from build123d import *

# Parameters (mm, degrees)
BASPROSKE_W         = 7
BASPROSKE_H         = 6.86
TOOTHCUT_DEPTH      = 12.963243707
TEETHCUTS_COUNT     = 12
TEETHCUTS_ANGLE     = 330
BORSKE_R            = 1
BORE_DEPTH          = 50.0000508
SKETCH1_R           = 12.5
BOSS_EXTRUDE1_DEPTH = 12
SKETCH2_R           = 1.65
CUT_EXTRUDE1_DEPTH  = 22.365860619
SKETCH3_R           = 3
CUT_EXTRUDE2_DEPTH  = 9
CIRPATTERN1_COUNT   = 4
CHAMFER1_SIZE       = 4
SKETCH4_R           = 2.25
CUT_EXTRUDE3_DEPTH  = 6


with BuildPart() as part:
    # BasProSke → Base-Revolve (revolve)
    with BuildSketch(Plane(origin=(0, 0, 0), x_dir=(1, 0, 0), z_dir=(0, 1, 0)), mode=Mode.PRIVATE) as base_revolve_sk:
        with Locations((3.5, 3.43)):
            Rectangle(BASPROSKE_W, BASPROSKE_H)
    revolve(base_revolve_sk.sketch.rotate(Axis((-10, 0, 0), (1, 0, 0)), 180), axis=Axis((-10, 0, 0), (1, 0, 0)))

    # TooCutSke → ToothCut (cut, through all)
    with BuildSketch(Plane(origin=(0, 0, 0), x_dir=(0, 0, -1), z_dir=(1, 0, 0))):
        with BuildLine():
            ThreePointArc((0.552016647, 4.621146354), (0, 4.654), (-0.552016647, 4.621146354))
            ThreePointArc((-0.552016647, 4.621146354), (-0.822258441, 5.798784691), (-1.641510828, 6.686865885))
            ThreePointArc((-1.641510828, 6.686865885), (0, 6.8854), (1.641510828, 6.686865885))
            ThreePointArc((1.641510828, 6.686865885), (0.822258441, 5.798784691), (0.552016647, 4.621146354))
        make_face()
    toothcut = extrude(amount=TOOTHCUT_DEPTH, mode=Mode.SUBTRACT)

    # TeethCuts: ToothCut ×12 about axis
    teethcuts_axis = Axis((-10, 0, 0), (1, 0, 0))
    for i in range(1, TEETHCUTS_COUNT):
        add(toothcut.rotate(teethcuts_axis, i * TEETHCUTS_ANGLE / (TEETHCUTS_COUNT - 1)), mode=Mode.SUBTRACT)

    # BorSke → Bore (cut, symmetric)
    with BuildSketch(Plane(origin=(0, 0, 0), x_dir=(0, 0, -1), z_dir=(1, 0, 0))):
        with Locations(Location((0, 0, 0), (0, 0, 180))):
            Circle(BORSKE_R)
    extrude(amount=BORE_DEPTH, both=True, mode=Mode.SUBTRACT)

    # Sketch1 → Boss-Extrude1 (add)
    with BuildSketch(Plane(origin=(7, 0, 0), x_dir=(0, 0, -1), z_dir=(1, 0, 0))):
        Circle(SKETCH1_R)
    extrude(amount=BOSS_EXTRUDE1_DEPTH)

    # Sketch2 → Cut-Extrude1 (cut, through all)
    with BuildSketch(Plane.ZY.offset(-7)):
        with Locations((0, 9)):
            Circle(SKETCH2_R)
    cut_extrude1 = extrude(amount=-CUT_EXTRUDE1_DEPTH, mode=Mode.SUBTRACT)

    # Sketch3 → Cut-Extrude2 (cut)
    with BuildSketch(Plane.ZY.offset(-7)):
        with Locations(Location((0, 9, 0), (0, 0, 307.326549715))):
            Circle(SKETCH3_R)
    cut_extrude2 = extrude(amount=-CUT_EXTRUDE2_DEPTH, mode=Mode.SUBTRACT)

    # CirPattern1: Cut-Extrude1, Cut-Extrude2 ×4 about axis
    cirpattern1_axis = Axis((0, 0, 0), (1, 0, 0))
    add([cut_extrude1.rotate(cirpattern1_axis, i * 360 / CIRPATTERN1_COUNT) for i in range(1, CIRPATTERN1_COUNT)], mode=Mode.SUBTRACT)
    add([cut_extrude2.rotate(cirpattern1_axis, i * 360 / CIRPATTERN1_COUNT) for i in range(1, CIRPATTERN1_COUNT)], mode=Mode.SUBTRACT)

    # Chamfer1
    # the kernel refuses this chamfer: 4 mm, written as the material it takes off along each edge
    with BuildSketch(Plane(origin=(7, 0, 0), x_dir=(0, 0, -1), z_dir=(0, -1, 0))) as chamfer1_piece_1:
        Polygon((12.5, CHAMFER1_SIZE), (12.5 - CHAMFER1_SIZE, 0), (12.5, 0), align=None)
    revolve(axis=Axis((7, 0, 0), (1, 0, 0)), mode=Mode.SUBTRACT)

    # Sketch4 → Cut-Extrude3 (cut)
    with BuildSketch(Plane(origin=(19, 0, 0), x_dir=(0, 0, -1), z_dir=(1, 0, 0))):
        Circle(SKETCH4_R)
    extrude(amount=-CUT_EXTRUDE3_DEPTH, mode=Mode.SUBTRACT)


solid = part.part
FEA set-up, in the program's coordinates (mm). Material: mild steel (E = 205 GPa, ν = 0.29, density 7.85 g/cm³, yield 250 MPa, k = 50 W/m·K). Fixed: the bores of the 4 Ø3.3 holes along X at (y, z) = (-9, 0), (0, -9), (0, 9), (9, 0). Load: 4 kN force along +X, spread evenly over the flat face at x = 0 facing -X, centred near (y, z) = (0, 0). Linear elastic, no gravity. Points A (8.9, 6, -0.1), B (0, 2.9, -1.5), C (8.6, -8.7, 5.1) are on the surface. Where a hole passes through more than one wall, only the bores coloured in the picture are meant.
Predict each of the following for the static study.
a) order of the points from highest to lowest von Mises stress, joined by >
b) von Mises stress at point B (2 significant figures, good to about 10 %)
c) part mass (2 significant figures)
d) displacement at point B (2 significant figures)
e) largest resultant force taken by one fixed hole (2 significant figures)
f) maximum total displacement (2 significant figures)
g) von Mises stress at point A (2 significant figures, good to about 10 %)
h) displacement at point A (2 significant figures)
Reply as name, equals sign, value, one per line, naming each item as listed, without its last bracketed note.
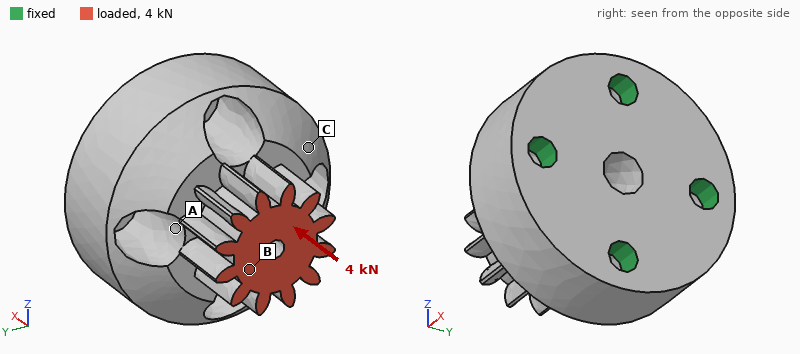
order of the points from highest to lowest von Mises stress, joined by > = B > A > C
von Mises stress at point B = 41 MPa
part mass = 39 g
displacement at point B = 3.5 µm
largest resultant force taken by one fixed hole = 1.0 kN
maximum total displacement = 3.6 µm
von Mises stress at point A = 21 MPa
displacement at point A = 1.9 µm
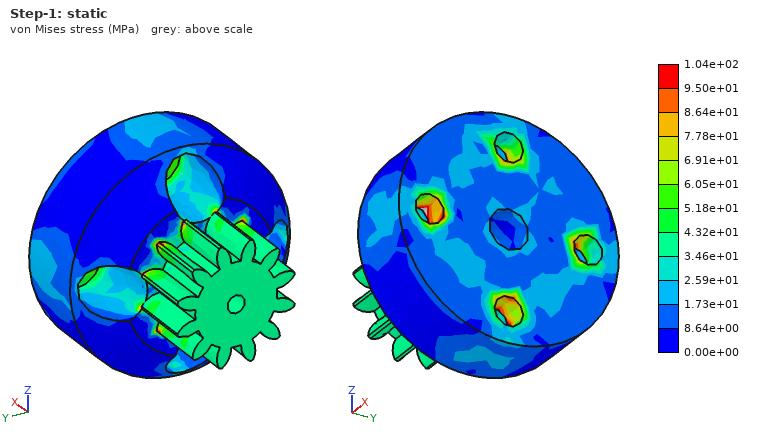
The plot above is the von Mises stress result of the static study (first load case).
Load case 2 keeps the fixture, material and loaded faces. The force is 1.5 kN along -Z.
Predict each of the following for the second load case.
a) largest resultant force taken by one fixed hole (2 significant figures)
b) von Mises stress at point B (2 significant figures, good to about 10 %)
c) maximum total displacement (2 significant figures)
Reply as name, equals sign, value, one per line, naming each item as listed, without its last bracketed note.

largest resultant force taken by one fixed hole = 1.4 kN
von Mises stress at point B = 32 MPa
maximum total displacement = 10.0 µm
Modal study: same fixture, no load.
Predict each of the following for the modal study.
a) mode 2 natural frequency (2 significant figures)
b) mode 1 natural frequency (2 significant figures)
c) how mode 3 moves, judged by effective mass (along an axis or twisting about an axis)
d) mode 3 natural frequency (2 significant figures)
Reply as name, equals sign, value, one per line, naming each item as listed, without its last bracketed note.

mode 2 natural frequency = 29 kHz
mode 1 natural frequency = 29 kHz
how mode 3 moves, judged by effective mass = along X
mode 3 natural frequency = 48 kHz
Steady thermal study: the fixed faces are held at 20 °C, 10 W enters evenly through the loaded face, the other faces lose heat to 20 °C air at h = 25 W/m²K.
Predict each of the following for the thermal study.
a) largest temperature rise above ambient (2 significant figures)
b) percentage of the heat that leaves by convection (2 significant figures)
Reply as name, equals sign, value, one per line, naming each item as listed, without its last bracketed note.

largest temperature rise above ambient = 26 K
percentage of the heat that leaves by convection = 4.8 %
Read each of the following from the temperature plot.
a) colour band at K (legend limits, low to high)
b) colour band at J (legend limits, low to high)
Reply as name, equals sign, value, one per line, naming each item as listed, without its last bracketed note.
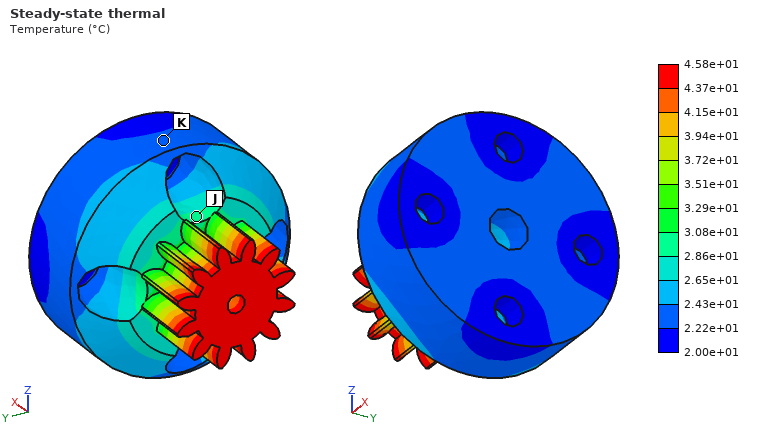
colour band at K = 2.22e+01 to 2.43e+01 °C
colour band at J = 2.86e+01 to 3.08e+01 °C
